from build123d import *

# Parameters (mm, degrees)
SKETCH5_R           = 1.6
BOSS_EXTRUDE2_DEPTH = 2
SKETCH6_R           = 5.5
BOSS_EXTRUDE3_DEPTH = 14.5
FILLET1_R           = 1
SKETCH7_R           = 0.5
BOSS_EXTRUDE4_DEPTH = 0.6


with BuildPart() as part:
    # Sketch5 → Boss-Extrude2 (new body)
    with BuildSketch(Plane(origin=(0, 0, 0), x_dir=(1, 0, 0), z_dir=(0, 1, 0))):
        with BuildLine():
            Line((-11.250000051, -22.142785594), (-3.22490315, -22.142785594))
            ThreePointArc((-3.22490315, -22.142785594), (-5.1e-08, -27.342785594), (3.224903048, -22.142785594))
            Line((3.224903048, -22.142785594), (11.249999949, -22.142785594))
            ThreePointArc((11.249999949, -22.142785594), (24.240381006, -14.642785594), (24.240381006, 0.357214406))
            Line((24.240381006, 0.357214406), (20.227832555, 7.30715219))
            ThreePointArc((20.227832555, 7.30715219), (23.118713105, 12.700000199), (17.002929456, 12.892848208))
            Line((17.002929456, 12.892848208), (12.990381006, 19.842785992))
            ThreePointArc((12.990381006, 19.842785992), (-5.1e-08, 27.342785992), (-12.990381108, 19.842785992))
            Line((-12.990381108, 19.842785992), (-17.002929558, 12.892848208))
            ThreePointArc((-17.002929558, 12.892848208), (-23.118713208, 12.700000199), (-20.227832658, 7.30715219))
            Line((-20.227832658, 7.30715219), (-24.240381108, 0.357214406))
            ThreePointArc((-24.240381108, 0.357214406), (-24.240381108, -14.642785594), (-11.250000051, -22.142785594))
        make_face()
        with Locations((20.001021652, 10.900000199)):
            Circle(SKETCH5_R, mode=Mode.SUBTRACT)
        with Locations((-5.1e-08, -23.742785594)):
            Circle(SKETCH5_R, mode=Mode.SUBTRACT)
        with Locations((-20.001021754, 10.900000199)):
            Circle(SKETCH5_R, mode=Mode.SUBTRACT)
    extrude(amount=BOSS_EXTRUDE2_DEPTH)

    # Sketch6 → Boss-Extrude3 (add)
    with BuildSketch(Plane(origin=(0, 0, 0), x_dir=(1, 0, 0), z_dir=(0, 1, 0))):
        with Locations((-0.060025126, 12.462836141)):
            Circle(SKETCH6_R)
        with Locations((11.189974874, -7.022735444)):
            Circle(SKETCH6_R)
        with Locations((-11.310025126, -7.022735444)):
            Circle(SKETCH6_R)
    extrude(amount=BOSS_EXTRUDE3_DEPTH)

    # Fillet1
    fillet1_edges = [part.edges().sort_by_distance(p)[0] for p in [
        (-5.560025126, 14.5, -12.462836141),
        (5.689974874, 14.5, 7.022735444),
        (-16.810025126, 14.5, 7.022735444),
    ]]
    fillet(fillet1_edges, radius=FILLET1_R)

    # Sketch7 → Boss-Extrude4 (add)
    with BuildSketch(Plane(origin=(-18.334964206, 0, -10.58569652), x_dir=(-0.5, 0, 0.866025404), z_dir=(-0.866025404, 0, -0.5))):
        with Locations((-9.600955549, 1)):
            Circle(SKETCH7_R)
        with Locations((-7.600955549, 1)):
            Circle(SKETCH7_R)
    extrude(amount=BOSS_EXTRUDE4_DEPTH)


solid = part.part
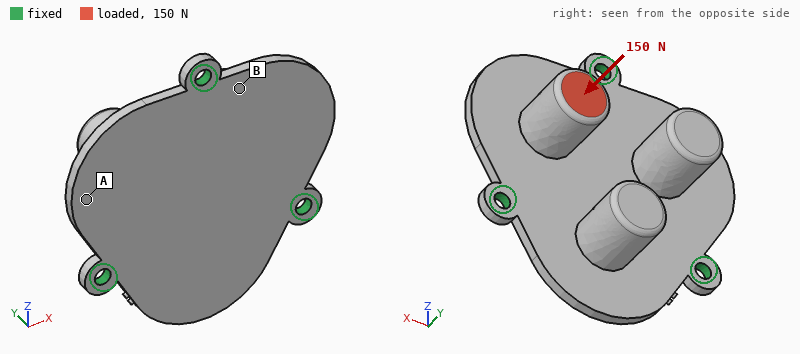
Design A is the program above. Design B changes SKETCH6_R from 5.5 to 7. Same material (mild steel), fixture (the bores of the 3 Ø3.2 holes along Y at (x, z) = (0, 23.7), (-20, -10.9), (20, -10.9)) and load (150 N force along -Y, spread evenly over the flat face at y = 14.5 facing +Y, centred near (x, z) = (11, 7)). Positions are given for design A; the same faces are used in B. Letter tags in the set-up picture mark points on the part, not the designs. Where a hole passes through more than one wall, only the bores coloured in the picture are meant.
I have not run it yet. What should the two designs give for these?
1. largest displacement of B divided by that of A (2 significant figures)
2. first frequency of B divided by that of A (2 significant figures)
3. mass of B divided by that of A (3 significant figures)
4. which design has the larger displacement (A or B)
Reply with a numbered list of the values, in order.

1. 0.79
2. 0.97
3. 1.29
4. A
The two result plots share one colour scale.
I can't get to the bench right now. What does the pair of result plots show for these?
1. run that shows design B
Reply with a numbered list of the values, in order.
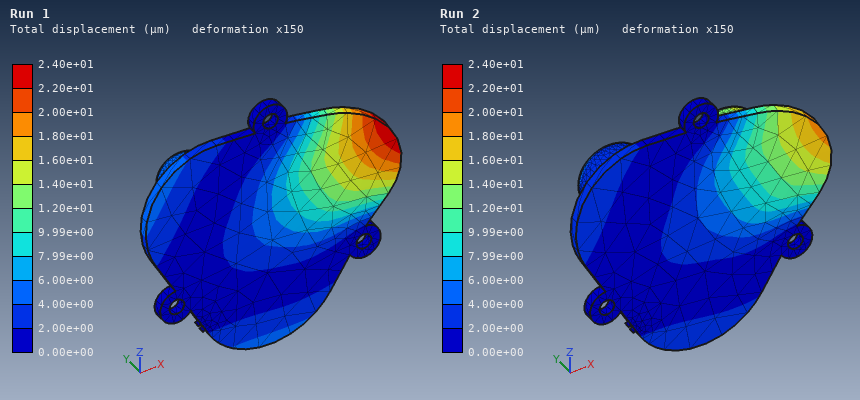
1. Run 2
